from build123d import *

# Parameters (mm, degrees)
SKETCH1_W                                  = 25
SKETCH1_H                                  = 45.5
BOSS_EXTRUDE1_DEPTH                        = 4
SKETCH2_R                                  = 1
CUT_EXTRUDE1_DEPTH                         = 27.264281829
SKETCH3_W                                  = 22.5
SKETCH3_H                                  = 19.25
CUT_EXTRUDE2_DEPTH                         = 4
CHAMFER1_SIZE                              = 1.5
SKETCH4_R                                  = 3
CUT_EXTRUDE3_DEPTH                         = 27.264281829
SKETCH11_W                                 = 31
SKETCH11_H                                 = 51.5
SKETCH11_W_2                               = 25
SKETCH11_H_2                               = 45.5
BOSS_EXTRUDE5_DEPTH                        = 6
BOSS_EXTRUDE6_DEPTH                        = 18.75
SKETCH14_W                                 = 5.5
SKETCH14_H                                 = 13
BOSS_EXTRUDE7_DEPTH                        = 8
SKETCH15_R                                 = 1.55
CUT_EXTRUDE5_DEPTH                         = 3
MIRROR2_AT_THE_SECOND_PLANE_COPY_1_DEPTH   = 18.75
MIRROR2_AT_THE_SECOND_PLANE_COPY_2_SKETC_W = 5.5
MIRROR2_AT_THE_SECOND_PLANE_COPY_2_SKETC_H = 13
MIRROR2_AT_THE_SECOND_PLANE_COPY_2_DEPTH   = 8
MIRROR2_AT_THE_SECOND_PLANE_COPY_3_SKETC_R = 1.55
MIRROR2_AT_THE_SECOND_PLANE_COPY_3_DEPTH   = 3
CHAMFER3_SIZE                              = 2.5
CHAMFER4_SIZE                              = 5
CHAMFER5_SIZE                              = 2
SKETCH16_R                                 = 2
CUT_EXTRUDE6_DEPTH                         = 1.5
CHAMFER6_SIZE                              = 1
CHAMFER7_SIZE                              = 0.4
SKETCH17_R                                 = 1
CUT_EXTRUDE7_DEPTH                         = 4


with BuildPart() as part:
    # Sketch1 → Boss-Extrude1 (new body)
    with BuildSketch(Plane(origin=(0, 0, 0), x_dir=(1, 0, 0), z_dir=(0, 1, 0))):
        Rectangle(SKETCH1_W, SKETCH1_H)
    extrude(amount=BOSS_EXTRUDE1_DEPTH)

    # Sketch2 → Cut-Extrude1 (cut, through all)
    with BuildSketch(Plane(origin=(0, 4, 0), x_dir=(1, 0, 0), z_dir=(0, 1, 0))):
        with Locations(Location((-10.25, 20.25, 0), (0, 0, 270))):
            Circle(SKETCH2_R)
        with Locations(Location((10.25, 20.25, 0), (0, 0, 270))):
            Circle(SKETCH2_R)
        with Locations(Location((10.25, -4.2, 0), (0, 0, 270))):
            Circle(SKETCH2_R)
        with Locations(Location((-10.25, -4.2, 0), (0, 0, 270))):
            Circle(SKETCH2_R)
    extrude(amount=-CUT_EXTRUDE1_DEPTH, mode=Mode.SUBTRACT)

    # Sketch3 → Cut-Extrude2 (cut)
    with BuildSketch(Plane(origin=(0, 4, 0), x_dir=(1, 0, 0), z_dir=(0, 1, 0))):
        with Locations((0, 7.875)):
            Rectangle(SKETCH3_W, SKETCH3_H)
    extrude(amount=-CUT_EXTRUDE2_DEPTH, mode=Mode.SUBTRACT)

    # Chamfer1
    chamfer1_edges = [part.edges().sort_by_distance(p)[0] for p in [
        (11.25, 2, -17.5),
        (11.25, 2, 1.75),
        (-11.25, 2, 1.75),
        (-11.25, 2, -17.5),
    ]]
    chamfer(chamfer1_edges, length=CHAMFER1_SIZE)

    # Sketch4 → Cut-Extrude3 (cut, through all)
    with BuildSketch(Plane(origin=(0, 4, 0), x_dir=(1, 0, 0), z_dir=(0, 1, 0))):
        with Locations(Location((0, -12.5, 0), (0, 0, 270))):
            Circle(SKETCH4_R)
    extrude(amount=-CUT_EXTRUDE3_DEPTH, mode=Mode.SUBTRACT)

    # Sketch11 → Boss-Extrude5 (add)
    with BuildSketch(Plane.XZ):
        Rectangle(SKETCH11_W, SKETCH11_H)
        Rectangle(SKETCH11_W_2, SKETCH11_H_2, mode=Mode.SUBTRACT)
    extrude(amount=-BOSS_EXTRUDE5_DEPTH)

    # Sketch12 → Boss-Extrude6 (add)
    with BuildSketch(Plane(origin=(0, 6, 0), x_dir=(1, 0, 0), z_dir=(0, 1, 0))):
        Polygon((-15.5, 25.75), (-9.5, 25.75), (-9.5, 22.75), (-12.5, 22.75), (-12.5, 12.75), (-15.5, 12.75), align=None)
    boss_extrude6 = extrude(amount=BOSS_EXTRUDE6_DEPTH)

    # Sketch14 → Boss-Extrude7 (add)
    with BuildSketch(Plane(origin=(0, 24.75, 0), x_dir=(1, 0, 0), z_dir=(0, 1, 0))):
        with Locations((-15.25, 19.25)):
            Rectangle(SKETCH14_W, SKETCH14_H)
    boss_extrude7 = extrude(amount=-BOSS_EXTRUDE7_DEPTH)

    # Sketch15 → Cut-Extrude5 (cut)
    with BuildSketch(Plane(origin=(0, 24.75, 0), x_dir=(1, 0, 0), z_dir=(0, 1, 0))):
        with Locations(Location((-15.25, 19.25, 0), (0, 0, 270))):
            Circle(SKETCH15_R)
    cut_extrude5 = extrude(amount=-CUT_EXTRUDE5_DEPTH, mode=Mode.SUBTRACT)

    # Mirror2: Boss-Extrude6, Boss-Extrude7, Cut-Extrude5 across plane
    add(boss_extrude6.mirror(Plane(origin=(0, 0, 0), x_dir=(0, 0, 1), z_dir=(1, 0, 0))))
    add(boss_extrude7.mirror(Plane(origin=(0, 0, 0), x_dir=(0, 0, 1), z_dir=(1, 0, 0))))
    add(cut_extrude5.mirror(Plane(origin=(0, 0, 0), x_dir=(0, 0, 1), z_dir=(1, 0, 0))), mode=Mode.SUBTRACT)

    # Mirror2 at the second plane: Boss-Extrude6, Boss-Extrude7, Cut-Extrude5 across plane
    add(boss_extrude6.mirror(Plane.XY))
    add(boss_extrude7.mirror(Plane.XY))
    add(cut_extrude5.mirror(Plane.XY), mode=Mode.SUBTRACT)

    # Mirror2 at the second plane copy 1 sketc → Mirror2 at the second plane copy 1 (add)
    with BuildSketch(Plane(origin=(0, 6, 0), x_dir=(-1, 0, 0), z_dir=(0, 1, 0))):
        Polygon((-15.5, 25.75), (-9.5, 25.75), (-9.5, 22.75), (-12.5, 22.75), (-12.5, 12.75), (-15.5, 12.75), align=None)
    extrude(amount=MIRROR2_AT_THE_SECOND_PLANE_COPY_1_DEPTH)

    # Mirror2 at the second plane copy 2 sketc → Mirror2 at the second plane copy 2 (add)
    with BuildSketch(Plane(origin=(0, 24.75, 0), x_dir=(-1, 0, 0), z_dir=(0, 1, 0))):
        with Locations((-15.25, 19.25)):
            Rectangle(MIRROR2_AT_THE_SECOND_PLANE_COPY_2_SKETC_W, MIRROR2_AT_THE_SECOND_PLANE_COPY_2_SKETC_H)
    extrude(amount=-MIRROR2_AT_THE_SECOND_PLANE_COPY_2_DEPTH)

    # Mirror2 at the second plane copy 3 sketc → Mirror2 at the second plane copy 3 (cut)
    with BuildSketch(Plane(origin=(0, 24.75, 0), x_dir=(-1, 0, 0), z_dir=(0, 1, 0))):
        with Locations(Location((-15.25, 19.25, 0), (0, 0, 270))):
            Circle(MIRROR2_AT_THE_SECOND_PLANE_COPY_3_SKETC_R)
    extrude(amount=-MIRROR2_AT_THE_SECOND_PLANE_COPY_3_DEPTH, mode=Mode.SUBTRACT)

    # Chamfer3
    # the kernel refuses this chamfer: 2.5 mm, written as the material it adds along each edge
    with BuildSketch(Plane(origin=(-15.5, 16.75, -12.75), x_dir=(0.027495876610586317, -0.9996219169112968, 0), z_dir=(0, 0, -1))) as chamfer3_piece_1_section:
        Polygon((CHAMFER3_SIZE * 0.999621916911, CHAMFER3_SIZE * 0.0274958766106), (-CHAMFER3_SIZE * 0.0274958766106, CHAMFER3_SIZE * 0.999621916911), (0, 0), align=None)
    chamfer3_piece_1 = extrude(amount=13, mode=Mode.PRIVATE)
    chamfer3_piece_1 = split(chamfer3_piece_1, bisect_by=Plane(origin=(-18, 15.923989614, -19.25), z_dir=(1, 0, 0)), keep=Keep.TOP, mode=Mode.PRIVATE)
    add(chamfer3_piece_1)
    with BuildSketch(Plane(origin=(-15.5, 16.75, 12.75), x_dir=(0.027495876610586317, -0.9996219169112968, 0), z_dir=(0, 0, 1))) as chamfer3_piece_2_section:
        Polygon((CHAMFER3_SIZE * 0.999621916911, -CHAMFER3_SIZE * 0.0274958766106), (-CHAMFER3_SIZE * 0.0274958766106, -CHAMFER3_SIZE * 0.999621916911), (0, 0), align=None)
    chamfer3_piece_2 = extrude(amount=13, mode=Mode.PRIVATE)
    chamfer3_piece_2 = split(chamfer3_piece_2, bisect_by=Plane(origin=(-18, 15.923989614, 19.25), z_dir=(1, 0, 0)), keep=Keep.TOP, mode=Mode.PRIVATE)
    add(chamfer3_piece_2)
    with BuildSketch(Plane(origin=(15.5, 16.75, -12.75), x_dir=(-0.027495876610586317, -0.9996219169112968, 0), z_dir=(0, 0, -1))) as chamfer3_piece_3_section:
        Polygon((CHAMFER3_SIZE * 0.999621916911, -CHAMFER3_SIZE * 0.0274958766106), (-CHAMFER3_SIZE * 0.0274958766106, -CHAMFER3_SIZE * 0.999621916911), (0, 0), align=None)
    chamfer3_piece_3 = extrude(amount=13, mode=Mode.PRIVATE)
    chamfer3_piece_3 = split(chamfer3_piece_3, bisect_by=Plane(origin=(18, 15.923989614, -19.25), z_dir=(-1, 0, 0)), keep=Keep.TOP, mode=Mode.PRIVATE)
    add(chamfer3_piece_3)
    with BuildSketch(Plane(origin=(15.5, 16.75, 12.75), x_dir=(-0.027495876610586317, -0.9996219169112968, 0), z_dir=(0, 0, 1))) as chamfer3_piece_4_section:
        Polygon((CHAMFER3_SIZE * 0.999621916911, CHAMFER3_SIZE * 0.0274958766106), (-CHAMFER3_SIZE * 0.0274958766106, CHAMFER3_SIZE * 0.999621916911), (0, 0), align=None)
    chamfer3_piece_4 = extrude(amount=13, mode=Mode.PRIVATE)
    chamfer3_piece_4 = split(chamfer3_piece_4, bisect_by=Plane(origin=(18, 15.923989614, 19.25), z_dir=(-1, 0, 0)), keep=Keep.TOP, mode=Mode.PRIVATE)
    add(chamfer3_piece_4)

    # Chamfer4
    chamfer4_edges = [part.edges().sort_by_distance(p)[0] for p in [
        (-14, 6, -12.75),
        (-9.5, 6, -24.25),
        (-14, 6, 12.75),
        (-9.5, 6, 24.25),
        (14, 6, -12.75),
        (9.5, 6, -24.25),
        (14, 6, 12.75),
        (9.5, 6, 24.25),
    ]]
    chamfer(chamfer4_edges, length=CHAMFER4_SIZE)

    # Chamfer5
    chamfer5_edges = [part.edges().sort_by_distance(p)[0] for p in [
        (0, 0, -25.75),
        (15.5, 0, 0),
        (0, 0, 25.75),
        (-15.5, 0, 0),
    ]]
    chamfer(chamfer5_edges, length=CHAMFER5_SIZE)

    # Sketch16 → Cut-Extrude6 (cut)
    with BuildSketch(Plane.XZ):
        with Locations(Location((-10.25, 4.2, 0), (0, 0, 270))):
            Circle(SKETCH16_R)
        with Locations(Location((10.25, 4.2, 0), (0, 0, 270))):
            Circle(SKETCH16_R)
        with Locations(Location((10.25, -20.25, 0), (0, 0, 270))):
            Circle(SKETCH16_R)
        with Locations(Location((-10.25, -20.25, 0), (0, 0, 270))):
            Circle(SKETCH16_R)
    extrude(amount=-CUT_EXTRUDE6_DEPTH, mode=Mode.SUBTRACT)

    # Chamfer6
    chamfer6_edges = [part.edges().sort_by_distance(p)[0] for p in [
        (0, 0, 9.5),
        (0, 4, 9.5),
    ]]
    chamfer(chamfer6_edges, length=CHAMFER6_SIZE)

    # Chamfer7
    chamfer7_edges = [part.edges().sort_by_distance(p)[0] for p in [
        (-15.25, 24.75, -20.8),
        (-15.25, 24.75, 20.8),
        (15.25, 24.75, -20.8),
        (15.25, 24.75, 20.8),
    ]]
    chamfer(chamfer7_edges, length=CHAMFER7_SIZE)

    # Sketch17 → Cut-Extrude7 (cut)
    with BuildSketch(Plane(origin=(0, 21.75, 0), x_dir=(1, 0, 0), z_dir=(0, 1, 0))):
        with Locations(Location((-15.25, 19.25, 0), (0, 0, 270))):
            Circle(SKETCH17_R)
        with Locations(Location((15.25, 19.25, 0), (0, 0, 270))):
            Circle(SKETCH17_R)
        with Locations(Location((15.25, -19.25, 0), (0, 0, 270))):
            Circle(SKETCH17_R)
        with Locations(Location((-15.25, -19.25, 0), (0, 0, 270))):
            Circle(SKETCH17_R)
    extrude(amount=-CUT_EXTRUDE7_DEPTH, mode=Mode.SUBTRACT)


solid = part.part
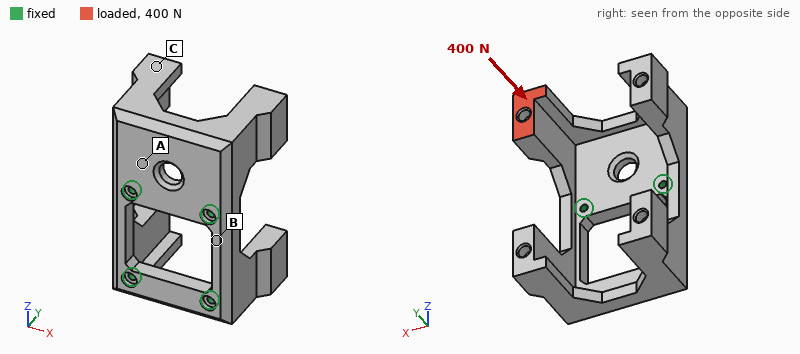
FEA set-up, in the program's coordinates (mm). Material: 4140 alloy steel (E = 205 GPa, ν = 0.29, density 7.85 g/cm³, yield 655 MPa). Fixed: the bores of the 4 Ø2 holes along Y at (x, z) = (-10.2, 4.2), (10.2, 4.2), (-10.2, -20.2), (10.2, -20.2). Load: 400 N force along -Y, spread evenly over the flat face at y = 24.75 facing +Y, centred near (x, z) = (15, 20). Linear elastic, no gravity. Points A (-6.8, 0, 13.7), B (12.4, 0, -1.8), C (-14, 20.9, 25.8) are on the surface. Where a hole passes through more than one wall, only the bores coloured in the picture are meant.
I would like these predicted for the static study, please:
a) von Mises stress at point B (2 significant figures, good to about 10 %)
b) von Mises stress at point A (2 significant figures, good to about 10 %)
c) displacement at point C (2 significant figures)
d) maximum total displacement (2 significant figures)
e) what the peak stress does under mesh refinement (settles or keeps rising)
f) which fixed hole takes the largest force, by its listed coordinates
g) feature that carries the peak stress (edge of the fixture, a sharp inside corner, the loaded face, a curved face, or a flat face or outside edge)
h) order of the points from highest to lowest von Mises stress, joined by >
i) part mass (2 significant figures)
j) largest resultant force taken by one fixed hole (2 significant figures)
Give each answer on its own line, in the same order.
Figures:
60 MPa
30 MPa
32 µm
89 µm
keeps rising
(10.2, 4.2)
edge of the fixture
B > A > C
78 g
540 N
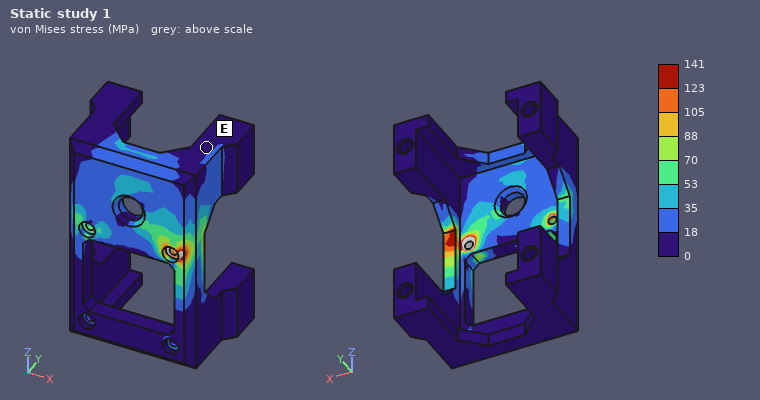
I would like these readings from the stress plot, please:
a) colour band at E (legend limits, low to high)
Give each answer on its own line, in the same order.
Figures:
0 to 18 MPa
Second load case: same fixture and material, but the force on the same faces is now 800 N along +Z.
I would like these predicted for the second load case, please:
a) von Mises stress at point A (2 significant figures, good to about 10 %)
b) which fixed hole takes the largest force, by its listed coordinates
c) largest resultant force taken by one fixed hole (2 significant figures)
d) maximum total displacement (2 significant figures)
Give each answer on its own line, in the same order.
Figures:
89 MPa
(10.2, 4.2)
550 N
0.28 mm
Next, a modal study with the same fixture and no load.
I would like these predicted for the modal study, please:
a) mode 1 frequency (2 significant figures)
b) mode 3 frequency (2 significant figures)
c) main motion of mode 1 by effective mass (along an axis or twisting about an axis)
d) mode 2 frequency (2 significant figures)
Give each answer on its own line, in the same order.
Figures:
2700 Hz
5000 Hz
along Y
3200 Hz
